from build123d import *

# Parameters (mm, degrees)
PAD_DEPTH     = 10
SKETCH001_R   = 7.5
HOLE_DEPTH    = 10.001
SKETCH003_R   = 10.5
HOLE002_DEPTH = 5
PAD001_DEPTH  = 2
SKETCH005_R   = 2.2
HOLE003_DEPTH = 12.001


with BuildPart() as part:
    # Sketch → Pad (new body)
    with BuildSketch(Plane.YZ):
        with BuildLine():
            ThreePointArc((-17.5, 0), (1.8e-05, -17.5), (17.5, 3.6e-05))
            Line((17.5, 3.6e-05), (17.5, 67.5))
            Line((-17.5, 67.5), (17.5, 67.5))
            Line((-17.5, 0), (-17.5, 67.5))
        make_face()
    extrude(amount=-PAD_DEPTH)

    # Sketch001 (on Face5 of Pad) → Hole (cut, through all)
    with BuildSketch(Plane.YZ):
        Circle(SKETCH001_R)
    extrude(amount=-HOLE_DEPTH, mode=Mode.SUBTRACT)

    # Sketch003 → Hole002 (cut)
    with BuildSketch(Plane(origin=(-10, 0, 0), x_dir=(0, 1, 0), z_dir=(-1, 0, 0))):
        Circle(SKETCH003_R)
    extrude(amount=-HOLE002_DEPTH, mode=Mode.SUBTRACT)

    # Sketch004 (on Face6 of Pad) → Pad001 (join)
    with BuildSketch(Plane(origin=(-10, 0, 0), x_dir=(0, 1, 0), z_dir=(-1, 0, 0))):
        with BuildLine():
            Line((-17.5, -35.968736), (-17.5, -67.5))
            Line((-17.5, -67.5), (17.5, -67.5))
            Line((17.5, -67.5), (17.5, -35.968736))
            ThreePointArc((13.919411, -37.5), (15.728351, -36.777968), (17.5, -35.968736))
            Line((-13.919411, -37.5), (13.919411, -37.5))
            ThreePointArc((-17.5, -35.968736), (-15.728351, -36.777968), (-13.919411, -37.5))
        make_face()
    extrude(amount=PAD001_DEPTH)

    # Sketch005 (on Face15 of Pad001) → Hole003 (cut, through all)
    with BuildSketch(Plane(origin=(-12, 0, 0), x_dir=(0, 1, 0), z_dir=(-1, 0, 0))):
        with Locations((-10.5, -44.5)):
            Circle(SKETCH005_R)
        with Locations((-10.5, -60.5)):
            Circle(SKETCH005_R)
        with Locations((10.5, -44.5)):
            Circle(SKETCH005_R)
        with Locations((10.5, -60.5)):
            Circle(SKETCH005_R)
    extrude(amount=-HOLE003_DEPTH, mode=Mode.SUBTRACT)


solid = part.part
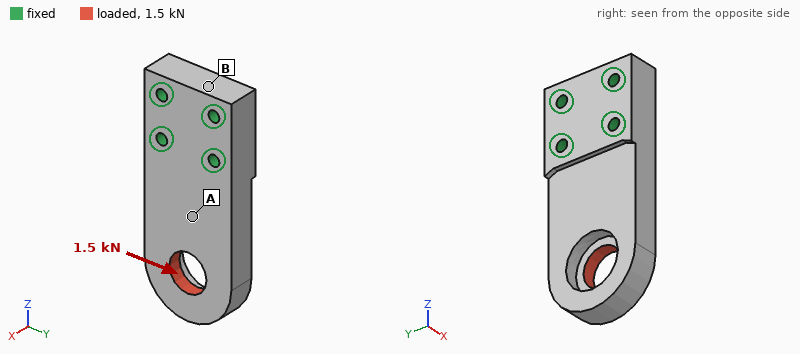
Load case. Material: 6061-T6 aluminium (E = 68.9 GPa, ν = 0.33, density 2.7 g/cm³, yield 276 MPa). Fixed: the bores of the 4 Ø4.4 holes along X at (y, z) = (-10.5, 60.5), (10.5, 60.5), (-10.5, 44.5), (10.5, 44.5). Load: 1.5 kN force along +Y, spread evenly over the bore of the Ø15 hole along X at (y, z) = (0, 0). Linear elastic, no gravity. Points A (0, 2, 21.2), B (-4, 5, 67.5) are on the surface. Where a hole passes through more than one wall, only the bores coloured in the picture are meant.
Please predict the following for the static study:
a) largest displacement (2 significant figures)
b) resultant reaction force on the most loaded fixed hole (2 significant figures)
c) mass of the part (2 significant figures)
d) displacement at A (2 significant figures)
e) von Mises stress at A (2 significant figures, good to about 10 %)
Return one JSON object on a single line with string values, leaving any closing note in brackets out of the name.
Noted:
{"largest displacement": "46 µm", "resultant reaction force on the most loaded fixed hole": "2.6 kN", "mass of the part": "73 g", "displacement at A": "11 µm", "von Mises stress at A": "18 MPa"}
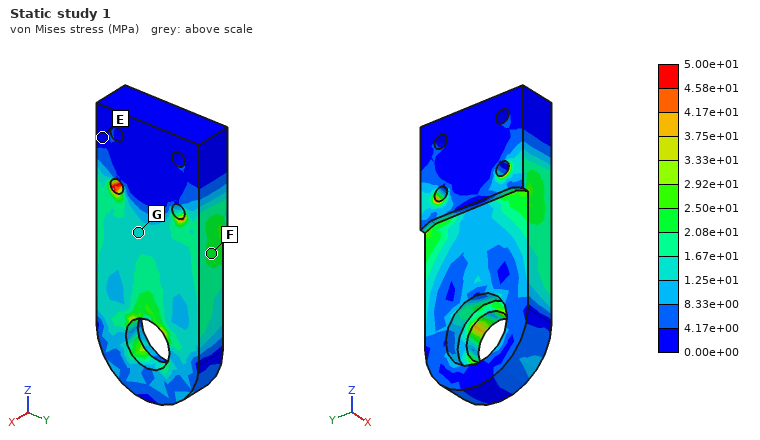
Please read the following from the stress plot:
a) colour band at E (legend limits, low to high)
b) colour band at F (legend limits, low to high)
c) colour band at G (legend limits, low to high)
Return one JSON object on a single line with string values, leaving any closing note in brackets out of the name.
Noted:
{"colour band at E": "0.00e+00 to 4.17e+00 MPa", "colour band at F": "2.08e+01 to 2.50e+01 MPa", "colour band at G": "1.25e+01 to 1.67e+01 MPa"}
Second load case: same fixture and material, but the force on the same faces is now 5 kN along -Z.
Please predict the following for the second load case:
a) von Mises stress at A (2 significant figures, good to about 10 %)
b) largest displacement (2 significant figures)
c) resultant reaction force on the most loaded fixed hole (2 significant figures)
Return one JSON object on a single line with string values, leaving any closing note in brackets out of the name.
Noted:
{"von Mises stress at A": "33 MPa", "largest displacement": "0.12 mm", "resultant reaction force on the most loaded fixed hole": "2.2 kN"}
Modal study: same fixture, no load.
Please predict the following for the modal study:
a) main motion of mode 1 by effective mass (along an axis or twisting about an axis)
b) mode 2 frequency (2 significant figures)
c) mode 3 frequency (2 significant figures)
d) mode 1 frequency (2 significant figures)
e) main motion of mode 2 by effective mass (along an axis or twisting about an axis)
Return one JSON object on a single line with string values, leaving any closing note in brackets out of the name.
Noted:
{"main motion of mode 1 by effective mass": "along X", "mode 2 frequency": "7000 Hz", "mode 3 frequency": "8000 Hz", "mode 1 frequency": "2800 Hz", "main motion of mode 2 by effective mass": "along Y"}
